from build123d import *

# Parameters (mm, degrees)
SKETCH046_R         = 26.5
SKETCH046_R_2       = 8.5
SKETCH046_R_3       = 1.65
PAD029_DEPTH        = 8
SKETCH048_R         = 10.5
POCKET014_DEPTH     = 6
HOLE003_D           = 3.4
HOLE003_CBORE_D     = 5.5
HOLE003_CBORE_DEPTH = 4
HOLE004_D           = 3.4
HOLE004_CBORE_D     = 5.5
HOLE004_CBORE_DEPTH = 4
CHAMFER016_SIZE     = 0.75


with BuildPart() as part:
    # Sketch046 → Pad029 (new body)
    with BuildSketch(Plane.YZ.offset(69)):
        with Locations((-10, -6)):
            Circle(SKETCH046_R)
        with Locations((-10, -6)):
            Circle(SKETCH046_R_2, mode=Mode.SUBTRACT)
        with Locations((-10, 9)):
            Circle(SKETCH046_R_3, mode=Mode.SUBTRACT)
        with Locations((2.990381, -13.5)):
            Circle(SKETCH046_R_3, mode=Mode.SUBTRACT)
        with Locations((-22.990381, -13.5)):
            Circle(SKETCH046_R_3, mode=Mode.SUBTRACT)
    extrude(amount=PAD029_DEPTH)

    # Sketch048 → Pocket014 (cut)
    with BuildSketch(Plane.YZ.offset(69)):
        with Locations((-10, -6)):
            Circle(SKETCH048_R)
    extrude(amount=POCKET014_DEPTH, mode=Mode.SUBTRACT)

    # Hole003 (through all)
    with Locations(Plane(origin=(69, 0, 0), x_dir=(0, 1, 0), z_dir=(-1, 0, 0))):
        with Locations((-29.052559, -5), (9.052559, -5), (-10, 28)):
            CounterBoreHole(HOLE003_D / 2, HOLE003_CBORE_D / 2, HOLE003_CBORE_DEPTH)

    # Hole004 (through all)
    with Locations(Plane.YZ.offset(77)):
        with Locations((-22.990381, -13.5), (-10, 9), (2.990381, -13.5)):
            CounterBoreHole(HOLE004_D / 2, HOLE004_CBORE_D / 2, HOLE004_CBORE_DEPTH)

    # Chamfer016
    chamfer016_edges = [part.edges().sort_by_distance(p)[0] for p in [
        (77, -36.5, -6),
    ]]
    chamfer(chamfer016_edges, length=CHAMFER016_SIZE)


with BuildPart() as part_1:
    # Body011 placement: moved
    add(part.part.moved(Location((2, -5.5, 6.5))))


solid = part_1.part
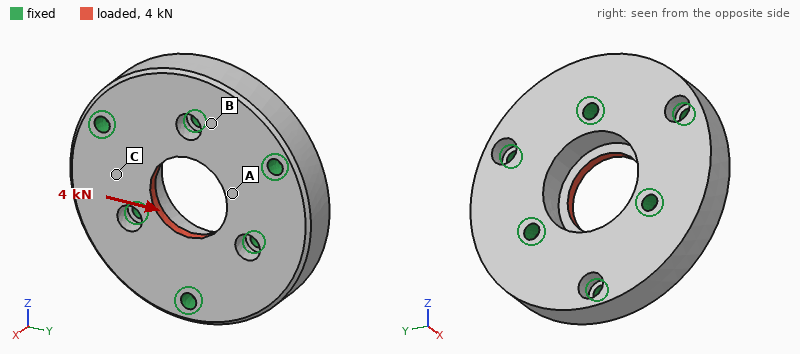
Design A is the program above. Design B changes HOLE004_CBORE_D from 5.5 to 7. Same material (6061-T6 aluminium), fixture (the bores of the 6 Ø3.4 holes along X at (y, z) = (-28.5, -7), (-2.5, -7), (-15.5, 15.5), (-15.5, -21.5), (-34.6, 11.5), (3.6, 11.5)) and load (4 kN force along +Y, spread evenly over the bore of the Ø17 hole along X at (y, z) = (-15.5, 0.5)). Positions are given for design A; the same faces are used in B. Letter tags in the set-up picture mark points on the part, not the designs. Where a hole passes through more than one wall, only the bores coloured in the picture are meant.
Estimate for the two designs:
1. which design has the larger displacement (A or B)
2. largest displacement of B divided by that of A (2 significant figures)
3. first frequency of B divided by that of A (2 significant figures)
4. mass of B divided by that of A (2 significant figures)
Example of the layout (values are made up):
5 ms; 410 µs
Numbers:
B; 1.2; 0.98; 0.99
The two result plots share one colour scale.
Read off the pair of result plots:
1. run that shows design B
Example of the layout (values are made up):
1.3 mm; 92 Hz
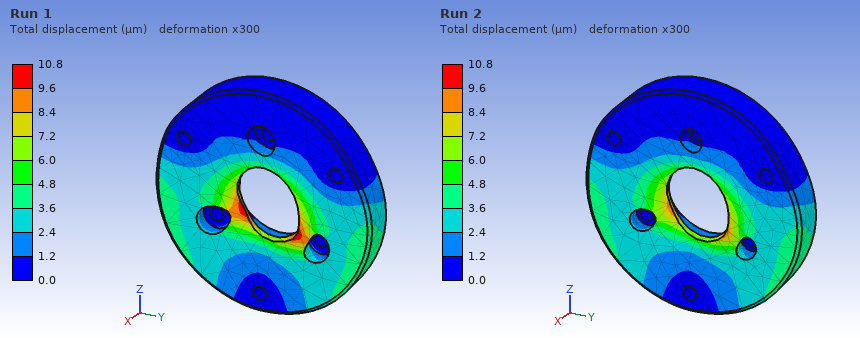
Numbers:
Run 1
